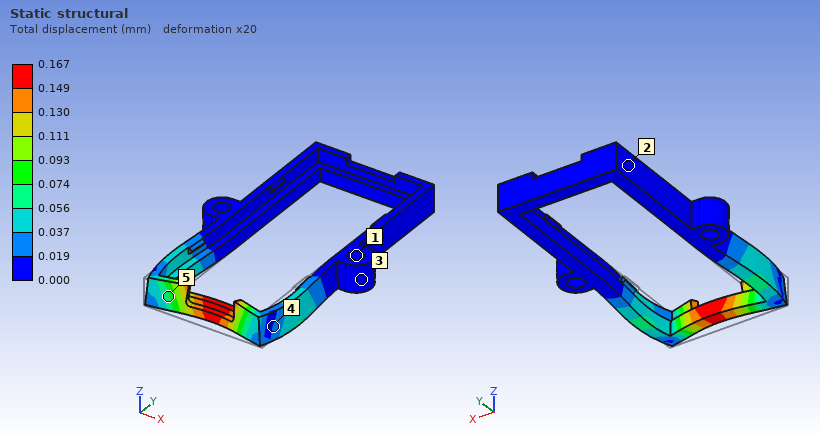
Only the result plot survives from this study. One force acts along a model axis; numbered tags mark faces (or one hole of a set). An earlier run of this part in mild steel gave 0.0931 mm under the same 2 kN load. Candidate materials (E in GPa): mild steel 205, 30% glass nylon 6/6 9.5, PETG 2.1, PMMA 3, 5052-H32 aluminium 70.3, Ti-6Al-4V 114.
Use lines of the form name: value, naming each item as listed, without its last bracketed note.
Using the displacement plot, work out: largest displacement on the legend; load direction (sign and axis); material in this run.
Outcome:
largest displacement on the legend: 0.167 mm
load direction: +Y
material in this run: Ti-6Al-4V
